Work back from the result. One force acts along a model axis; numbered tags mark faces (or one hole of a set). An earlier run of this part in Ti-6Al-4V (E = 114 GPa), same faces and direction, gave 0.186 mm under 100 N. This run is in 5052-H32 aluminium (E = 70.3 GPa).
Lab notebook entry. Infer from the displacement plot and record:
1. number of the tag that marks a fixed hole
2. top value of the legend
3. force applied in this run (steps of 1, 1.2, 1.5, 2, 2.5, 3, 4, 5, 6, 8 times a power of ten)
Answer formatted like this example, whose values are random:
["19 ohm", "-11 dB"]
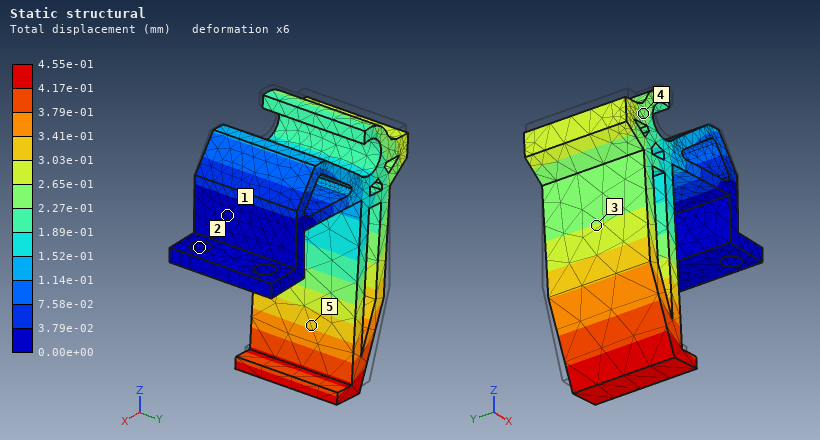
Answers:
["2", "4.55e-01 mm", "150 N"]
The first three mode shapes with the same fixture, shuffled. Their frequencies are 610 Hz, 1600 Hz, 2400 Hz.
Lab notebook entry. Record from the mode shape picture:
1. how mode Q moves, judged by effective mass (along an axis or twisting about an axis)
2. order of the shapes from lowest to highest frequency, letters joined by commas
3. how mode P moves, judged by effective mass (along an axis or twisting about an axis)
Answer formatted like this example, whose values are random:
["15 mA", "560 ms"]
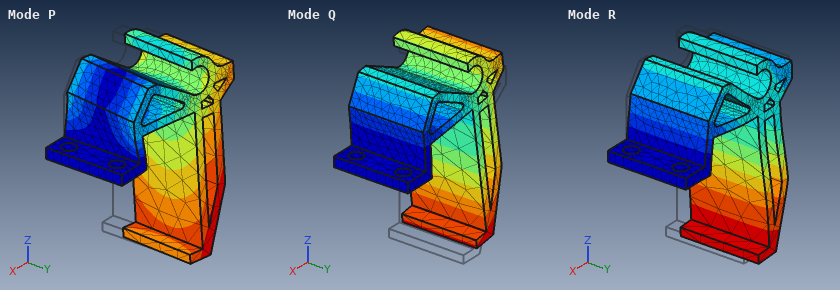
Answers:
["along Z", "Q, P, R", "along Y"]
